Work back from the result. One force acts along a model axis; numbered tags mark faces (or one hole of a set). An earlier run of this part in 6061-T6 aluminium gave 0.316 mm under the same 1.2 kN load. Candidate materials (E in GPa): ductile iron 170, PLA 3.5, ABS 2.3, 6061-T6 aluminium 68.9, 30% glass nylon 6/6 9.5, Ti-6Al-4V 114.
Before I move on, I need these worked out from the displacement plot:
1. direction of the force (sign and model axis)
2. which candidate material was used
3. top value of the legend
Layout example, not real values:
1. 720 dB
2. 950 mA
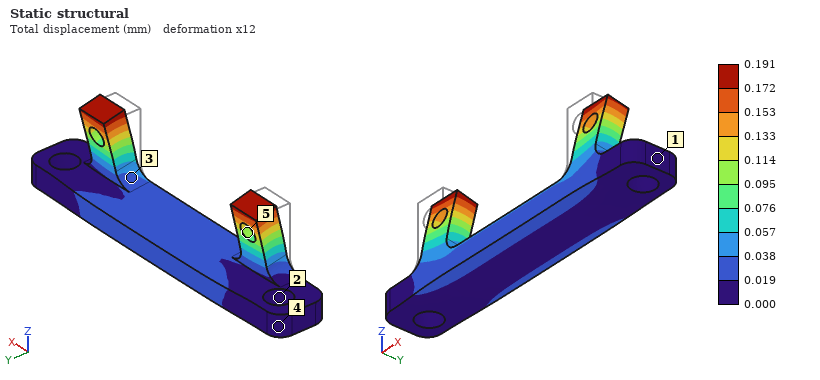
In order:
1. +Y
2. Ti-6Al-4V
3. 0.191 mm
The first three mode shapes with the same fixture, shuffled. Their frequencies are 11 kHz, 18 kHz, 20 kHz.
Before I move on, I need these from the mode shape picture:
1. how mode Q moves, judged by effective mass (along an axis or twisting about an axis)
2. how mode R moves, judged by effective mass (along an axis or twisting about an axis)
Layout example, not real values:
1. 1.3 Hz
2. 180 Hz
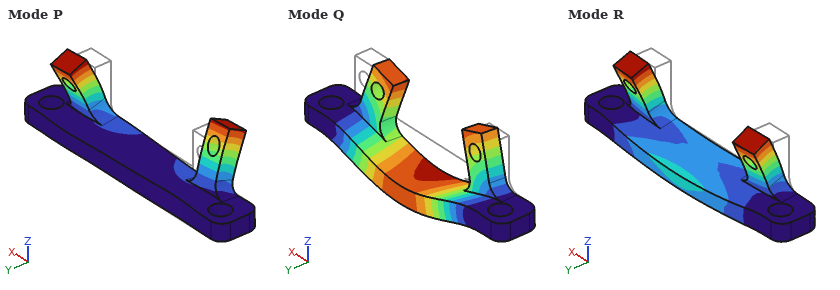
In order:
1. along Z
2. along Y
